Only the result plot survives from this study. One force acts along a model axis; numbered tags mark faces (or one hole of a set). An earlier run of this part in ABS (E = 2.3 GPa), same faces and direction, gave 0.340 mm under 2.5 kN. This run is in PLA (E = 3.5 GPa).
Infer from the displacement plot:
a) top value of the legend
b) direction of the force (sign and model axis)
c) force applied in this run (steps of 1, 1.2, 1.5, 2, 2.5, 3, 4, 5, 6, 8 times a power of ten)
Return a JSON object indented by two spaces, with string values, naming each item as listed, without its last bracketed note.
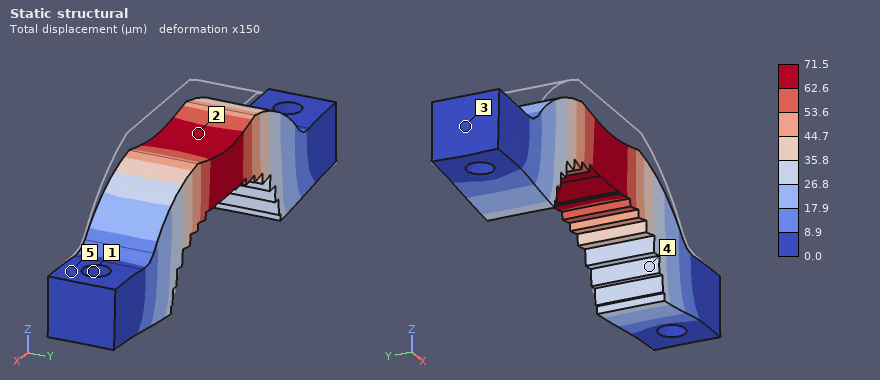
{
  "top value of the legend": "71.5 µm",
  "direction of the force": "-Z",
  "force applied in this run": "800 N"
}
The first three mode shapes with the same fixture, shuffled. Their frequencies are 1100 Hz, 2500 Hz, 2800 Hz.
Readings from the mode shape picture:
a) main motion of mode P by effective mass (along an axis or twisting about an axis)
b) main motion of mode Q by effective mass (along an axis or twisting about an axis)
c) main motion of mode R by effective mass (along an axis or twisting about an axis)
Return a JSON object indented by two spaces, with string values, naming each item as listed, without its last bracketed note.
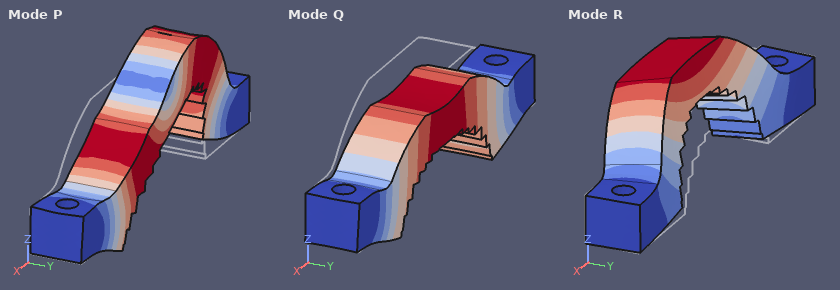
{
  "main motion of mode P by effective mass": "along X",
  "main motion of mode Q by effective mass": "along Z",
  "main motion of mode R by effective mass": "along Y"
}
